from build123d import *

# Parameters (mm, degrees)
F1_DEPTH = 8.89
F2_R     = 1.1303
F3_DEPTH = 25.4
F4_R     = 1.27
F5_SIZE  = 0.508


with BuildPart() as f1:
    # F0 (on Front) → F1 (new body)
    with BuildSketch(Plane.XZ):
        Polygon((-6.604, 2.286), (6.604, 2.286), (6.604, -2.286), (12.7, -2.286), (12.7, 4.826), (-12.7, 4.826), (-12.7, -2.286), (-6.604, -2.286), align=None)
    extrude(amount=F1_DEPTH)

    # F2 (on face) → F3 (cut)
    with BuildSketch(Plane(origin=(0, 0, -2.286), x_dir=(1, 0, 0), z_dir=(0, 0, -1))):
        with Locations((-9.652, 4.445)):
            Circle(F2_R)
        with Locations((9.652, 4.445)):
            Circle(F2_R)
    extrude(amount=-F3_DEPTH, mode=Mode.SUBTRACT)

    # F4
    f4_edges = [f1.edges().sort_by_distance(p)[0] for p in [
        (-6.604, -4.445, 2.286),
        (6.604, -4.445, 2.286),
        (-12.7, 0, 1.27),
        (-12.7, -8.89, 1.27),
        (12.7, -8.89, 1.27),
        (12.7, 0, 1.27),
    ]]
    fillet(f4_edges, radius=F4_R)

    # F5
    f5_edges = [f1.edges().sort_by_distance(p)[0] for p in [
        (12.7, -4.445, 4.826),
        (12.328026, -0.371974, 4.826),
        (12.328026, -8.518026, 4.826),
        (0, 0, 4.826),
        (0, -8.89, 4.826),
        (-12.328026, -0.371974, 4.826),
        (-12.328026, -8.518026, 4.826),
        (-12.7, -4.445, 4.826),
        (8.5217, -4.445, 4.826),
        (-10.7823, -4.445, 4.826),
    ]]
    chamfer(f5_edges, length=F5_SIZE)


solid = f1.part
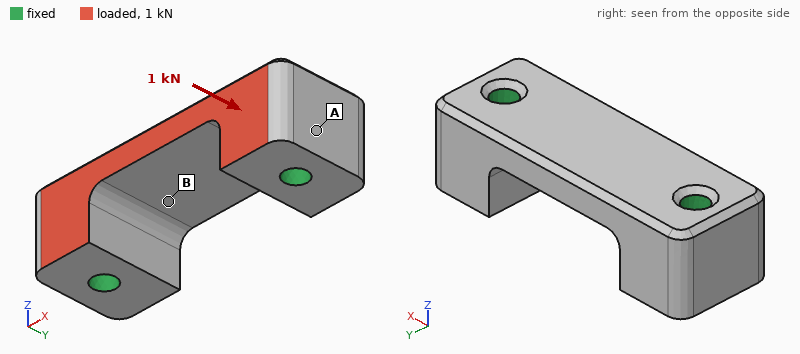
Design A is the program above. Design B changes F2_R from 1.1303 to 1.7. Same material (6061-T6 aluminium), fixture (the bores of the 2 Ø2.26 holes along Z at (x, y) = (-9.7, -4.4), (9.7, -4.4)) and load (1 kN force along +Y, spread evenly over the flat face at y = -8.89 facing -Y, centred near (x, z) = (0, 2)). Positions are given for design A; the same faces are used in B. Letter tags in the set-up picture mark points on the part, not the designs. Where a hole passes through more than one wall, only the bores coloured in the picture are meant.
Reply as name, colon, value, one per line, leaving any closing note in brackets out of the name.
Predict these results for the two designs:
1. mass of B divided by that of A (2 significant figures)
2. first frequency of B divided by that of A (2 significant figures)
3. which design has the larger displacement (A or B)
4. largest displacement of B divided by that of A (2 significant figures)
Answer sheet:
mass of B divided by that of A: 0.93
first frequency of B divided by that of A: 1.0
which design has the larger displacement: A
largest displacement of B divided by that of A: 0.82
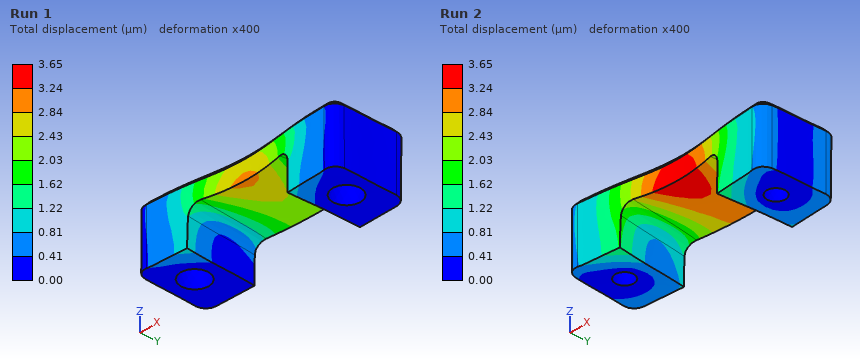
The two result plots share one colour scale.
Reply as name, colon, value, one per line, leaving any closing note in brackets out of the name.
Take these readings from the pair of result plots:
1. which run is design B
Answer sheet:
which run is design B: Run 1
